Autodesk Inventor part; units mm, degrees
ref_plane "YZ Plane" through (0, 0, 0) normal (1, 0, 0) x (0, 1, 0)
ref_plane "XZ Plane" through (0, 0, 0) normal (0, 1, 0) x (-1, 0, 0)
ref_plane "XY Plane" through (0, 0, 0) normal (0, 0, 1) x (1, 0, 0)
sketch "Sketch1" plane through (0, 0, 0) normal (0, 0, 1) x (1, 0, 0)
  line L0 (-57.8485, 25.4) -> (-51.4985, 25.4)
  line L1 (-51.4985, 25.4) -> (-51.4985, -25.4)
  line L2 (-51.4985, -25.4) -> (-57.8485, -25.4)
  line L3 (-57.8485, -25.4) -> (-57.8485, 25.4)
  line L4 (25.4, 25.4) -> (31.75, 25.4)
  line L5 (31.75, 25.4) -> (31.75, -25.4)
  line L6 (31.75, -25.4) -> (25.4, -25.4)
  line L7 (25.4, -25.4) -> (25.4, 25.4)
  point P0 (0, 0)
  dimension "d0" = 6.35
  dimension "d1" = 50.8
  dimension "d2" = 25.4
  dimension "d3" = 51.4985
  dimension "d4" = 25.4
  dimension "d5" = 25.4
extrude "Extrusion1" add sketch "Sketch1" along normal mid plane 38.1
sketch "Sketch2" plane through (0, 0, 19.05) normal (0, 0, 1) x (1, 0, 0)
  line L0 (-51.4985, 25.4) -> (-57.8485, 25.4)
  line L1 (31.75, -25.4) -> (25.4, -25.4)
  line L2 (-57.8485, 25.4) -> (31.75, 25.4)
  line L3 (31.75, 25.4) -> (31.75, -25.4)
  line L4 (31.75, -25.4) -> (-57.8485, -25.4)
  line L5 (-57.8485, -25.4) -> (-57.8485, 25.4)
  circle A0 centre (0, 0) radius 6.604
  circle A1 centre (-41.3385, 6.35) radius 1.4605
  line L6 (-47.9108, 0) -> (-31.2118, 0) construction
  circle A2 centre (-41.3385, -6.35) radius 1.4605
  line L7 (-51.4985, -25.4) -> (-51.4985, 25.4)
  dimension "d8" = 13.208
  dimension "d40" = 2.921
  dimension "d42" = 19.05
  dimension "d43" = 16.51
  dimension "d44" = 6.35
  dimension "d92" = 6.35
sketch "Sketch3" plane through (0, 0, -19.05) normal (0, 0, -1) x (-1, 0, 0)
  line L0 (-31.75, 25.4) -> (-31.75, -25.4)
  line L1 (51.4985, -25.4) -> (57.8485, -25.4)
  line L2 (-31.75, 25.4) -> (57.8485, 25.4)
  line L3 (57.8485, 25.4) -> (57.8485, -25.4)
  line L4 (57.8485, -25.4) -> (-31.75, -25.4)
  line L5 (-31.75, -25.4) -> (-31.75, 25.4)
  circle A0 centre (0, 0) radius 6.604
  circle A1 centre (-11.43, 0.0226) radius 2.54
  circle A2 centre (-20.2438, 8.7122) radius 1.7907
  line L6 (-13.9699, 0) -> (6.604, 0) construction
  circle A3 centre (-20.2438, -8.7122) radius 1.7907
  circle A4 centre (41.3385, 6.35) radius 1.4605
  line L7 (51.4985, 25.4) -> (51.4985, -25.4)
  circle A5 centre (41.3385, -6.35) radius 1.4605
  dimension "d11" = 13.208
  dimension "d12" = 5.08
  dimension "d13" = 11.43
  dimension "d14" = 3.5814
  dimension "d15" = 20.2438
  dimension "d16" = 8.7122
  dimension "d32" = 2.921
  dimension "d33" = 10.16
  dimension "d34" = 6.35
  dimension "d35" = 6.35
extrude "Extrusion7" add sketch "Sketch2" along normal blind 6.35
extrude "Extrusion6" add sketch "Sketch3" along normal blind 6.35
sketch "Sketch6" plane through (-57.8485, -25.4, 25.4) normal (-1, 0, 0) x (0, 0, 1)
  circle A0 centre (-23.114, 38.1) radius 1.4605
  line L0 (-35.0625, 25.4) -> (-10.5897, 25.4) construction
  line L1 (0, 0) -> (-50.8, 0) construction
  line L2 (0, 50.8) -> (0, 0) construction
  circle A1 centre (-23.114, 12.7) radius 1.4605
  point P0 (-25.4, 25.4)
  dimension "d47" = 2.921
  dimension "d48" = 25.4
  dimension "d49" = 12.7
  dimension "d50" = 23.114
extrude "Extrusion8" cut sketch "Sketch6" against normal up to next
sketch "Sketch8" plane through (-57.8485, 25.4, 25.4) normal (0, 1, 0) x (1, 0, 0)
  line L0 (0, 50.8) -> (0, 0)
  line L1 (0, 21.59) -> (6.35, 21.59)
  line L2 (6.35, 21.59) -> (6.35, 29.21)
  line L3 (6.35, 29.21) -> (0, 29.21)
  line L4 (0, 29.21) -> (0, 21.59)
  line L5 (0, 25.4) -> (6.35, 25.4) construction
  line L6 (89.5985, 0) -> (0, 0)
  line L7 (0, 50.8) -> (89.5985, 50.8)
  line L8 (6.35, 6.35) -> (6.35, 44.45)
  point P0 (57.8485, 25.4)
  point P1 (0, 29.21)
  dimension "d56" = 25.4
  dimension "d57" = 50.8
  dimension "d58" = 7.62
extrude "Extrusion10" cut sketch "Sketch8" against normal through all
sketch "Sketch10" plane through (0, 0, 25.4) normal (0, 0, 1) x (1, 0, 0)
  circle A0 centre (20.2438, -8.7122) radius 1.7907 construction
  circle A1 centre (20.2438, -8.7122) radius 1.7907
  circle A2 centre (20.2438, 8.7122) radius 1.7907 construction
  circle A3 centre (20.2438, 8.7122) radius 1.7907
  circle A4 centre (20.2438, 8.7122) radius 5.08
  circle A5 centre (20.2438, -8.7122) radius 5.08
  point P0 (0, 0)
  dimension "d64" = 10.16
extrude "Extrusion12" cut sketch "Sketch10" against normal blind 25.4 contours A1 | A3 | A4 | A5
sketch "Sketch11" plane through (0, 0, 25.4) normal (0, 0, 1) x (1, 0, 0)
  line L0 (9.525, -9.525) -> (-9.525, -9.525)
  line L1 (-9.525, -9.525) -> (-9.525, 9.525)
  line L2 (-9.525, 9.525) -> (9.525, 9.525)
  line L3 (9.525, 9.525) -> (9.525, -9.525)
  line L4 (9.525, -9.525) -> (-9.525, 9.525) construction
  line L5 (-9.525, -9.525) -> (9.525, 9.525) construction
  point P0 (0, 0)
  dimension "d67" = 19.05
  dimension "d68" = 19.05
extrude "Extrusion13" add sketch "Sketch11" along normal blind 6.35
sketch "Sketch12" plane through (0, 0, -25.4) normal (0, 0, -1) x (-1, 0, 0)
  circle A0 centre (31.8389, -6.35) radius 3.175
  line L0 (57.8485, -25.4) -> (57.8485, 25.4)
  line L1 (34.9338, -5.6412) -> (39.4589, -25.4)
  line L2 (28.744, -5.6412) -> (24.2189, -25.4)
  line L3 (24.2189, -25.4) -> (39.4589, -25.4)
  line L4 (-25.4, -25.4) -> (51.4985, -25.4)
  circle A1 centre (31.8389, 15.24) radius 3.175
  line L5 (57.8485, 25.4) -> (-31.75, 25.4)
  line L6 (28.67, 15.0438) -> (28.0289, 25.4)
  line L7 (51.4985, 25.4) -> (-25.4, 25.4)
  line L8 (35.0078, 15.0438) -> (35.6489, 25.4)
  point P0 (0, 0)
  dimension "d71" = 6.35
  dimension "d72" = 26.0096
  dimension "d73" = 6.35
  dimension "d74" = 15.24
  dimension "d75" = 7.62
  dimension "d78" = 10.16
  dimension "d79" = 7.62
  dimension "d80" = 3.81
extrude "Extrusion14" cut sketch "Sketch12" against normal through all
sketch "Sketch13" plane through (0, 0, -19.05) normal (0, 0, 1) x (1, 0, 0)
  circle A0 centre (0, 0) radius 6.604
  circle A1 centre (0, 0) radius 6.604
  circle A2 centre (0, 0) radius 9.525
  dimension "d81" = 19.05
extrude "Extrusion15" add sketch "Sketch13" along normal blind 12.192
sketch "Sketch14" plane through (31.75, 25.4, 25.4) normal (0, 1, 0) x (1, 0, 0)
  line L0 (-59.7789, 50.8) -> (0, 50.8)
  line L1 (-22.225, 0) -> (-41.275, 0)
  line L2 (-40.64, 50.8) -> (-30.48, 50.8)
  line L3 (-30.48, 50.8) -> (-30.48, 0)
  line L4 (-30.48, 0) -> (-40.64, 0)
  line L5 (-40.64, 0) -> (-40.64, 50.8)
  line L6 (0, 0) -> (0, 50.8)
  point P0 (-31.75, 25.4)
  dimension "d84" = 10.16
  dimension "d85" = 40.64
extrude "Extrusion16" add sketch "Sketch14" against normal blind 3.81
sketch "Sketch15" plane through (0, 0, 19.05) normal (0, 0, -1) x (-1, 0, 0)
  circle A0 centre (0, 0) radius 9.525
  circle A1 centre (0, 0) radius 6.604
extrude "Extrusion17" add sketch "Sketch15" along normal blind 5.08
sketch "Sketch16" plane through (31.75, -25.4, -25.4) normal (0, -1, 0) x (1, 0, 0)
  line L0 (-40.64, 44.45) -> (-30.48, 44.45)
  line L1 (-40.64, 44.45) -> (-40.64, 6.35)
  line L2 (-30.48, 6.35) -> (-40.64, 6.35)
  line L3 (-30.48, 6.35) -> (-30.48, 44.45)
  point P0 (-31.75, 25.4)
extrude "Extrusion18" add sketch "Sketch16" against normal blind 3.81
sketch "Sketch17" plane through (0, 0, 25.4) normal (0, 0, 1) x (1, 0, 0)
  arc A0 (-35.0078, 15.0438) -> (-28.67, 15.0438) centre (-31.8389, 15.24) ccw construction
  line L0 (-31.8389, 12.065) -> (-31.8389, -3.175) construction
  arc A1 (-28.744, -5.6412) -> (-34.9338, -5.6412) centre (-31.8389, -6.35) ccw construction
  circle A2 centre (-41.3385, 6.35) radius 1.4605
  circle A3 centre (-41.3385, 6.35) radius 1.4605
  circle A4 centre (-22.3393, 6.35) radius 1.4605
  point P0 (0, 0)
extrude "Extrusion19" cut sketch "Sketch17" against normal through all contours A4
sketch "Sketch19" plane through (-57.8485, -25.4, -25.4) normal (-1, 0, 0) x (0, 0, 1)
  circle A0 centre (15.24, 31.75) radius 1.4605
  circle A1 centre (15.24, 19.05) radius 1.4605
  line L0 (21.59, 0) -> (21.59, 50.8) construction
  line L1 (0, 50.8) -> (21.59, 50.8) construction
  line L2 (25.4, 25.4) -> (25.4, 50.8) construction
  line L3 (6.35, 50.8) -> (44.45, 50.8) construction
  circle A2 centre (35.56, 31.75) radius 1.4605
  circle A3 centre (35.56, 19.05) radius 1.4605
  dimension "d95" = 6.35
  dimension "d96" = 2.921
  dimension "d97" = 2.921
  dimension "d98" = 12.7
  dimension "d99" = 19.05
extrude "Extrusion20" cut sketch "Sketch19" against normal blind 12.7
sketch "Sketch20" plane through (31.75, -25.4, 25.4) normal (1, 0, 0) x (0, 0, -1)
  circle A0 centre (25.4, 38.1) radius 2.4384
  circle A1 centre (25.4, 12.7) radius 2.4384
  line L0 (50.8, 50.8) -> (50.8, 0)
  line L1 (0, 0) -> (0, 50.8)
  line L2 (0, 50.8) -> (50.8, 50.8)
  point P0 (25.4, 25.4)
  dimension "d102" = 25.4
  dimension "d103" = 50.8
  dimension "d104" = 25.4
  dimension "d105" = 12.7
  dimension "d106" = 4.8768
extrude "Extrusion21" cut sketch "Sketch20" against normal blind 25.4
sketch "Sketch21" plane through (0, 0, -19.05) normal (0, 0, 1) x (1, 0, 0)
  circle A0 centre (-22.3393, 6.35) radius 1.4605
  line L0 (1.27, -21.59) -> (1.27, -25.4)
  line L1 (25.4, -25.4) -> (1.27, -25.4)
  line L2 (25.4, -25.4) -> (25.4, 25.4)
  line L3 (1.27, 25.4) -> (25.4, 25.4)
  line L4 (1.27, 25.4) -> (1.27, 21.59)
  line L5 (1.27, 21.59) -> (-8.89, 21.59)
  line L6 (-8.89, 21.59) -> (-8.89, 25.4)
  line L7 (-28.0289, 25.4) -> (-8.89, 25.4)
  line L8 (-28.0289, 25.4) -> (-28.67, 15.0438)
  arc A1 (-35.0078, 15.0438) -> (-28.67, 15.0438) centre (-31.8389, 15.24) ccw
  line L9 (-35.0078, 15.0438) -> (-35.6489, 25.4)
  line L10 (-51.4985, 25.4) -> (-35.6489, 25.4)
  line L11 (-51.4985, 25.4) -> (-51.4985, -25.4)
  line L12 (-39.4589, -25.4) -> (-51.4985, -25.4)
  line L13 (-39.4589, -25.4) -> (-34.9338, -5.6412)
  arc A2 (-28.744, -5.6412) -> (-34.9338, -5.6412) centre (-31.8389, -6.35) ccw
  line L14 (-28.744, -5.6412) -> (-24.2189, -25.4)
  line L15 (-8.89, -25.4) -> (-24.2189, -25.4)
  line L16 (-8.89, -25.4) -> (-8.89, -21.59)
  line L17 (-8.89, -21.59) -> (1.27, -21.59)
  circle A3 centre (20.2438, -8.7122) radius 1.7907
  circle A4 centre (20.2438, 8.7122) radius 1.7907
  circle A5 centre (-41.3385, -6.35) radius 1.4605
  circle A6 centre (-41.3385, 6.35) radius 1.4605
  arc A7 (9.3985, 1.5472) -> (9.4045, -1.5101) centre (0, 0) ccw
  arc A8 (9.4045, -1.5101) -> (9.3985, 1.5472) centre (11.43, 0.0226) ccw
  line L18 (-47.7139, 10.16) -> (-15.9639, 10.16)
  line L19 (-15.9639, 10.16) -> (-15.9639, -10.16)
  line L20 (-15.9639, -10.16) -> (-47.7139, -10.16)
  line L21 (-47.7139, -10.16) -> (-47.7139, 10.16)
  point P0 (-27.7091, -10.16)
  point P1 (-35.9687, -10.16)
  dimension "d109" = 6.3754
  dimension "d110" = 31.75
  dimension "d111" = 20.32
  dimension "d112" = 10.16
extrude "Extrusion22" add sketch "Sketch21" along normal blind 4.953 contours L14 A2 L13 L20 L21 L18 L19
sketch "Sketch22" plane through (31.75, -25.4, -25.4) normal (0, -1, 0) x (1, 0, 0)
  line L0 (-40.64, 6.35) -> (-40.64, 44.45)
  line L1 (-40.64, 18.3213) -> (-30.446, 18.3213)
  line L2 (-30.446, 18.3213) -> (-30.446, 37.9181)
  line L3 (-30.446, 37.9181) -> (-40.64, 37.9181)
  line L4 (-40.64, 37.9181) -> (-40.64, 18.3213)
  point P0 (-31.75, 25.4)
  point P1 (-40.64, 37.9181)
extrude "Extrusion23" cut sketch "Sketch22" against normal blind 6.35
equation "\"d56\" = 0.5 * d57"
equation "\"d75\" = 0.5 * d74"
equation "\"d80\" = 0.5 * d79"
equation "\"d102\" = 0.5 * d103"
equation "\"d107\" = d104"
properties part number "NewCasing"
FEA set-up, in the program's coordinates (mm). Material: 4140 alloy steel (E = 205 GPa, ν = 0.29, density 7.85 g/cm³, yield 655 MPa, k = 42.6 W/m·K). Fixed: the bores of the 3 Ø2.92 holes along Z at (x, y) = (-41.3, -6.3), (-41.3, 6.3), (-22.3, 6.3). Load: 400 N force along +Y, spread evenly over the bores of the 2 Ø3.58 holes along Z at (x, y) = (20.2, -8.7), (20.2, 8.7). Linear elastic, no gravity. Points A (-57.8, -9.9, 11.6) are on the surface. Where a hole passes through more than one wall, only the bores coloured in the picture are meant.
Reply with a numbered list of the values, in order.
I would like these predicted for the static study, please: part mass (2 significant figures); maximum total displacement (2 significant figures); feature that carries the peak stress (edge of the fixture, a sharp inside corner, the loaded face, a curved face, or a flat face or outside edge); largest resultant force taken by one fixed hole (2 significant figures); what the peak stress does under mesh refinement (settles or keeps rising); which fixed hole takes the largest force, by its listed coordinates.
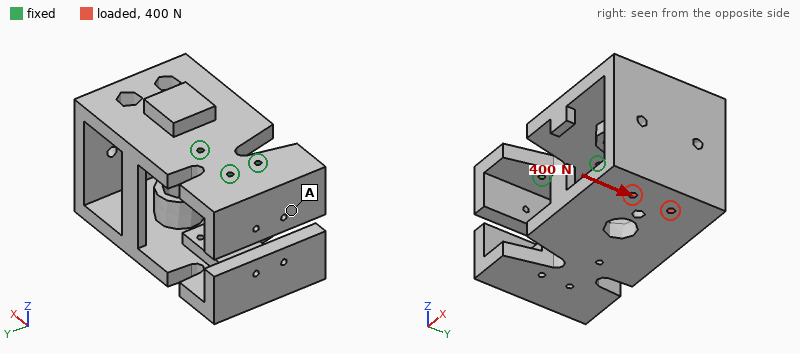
1. 650 g
2. 0.20 mm
3. edge of the fixture
4. 1.2 kN
5. keeps rising
6. (-22.3, 6.3)
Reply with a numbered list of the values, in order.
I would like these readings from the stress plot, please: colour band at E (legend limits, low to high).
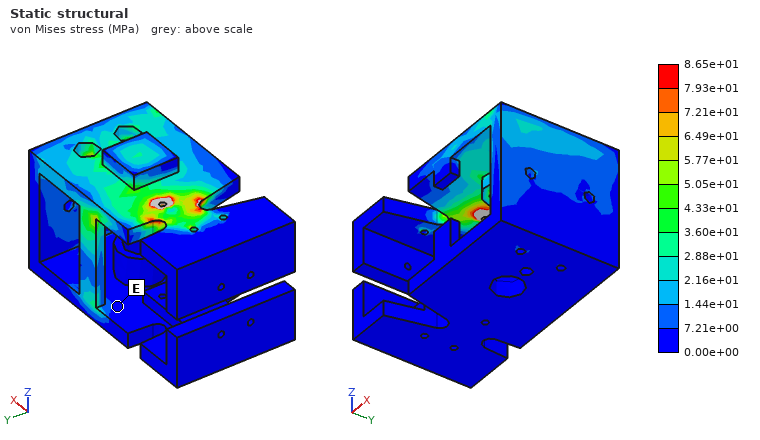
1. 0.00e+00 to 7.21e+00 MPa
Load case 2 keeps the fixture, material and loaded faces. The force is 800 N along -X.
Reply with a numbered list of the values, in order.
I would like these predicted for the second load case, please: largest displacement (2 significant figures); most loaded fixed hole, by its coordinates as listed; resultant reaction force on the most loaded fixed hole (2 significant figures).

1. 0.49 mm
2. (-22.3, 6.3)
3. 1.1 kN
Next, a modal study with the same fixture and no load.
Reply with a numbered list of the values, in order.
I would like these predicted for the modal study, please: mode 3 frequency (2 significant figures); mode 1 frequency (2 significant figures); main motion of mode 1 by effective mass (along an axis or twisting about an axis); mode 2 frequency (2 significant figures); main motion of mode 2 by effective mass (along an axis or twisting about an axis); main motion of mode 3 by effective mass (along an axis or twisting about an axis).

1. 710 Hz
2. 360 Hz
3. along X
4. 390 Hz
5. along Y
6. along Z
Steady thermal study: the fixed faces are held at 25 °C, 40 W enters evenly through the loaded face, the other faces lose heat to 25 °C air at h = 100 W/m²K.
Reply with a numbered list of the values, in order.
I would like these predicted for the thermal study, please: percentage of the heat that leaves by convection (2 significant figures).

1. 97 %
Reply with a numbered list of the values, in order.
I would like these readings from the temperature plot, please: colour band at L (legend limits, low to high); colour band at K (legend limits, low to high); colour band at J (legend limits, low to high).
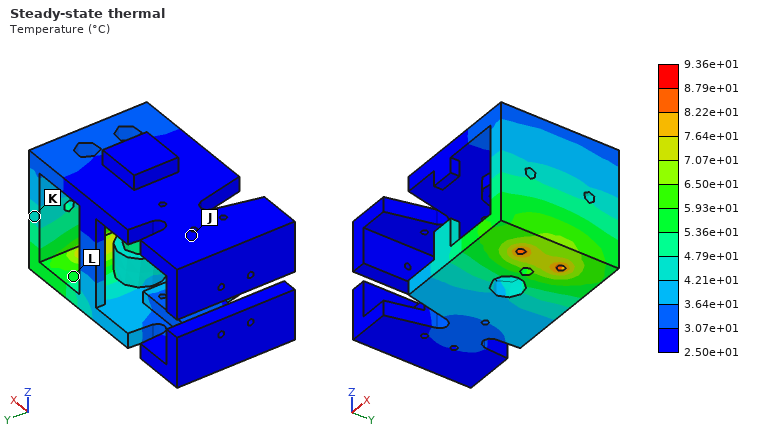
1. 5.36e+01 to 5.93e+01 °C
2. 4.21e+01 to 4.79e+01 °C
3. 2.50e+01 to 3.07e+01 °C
